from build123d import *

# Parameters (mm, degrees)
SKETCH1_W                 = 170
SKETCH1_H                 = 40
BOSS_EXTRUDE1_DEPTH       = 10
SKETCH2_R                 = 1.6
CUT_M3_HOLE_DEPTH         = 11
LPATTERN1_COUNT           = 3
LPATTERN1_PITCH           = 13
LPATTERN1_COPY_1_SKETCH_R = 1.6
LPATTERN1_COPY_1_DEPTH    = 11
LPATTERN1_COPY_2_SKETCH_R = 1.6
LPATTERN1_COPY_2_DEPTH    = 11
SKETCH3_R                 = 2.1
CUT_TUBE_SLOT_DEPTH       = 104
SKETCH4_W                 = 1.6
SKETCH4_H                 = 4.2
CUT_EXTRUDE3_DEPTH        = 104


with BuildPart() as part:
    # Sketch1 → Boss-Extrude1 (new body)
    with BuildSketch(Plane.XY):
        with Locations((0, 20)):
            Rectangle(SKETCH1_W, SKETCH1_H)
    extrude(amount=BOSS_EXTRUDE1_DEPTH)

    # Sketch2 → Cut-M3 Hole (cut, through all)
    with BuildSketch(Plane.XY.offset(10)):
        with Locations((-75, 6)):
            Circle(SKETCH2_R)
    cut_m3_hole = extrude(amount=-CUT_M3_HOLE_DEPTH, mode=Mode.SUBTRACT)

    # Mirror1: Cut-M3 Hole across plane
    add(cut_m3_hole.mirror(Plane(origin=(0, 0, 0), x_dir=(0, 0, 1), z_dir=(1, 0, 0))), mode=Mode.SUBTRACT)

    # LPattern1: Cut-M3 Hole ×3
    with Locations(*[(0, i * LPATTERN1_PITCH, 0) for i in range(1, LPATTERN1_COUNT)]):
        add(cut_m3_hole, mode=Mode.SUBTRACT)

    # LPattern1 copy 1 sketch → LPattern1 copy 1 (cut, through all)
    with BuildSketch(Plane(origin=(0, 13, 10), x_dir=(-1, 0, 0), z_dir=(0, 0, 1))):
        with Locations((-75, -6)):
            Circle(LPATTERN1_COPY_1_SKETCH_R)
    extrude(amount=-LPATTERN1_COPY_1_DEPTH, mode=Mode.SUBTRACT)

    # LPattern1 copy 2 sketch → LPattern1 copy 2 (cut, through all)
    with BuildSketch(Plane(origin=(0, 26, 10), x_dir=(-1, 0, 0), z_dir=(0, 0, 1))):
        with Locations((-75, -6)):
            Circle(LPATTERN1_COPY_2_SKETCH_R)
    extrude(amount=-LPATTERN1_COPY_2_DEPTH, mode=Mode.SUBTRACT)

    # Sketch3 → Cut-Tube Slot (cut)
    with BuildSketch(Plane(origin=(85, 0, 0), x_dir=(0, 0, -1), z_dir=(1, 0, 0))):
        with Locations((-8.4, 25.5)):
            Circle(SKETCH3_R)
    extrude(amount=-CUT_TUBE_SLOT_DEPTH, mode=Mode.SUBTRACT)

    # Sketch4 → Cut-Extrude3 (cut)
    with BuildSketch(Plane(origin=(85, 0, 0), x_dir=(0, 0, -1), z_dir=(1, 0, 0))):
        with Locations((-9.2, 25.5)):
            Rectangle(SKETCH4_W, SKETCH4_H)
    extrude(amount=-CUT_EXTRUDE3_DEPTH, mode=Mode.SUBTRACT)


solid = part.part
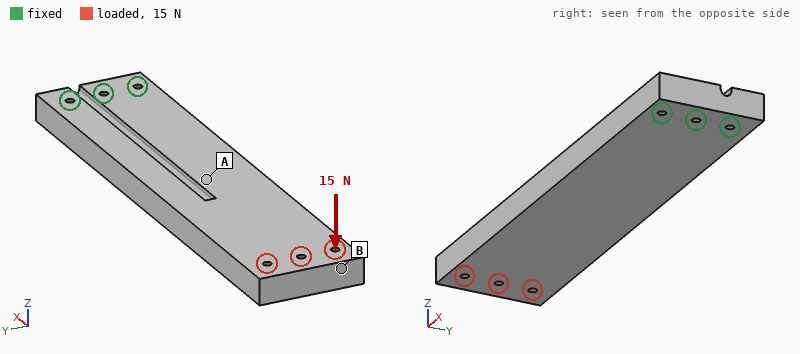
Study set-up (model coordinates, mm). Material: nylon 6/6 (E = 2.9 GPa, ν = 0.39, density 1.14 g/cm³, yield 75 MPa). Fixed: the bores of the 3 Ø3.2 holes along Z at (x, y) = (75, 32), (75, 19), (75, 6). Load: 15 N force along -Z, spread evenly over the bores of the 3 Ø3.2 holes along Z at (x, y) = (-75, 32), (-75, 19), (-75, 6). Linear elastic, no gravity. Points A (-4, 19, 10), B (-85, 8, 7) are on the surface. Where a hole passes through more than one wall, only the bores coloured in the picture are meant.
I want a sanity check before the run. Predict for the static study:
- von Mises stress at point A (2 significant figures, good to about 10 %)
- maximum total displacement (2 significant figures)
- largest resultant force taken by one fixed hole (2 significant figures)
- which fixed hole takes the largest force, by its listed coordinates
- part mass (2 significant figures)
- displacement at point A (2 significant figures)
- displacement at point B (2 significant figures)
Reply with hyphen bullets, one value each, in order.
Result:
- 1.7 MPa
- 2.0 mm
- 25 N
- (75, 19)
- 75 g
- 0.64 mm
- 2.0 mm
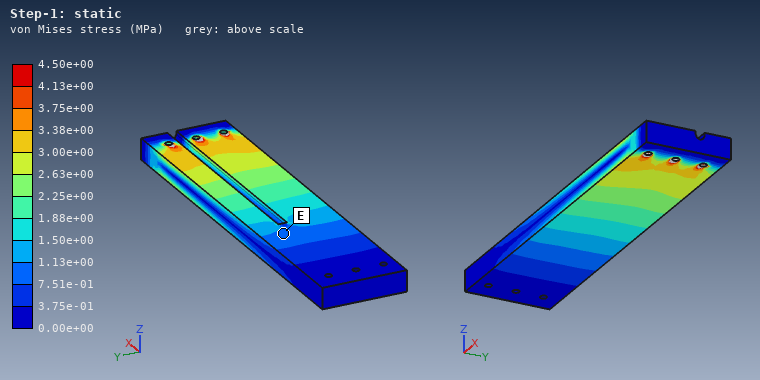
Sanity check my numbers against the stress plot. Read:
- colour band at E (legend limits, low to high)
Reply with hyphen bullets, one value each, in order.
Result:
- 7.51e-01 to 1.13e+00 MPa
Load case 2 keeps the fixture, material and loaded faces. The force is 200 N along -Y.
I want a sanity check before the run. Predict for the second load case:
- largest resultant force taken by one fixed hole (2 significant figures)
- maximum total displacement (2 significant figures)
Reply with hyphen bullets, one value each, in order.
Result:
- 1.1 kN
- 1.8 mm
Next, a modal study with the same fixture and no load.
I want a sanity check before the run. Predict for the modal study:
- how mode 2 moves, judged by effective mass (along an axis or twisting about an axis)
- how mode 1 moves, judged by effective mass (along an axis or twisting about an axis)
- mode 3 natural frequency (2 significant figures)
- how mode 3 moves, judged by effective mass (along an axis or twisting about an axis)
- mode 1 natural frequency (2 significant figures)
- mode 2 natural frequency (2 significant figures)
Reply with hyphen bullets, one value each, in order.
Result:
- along Y
- along Z
- 610 Hz
- along Z
- 99 Hz
- 370 Hz
